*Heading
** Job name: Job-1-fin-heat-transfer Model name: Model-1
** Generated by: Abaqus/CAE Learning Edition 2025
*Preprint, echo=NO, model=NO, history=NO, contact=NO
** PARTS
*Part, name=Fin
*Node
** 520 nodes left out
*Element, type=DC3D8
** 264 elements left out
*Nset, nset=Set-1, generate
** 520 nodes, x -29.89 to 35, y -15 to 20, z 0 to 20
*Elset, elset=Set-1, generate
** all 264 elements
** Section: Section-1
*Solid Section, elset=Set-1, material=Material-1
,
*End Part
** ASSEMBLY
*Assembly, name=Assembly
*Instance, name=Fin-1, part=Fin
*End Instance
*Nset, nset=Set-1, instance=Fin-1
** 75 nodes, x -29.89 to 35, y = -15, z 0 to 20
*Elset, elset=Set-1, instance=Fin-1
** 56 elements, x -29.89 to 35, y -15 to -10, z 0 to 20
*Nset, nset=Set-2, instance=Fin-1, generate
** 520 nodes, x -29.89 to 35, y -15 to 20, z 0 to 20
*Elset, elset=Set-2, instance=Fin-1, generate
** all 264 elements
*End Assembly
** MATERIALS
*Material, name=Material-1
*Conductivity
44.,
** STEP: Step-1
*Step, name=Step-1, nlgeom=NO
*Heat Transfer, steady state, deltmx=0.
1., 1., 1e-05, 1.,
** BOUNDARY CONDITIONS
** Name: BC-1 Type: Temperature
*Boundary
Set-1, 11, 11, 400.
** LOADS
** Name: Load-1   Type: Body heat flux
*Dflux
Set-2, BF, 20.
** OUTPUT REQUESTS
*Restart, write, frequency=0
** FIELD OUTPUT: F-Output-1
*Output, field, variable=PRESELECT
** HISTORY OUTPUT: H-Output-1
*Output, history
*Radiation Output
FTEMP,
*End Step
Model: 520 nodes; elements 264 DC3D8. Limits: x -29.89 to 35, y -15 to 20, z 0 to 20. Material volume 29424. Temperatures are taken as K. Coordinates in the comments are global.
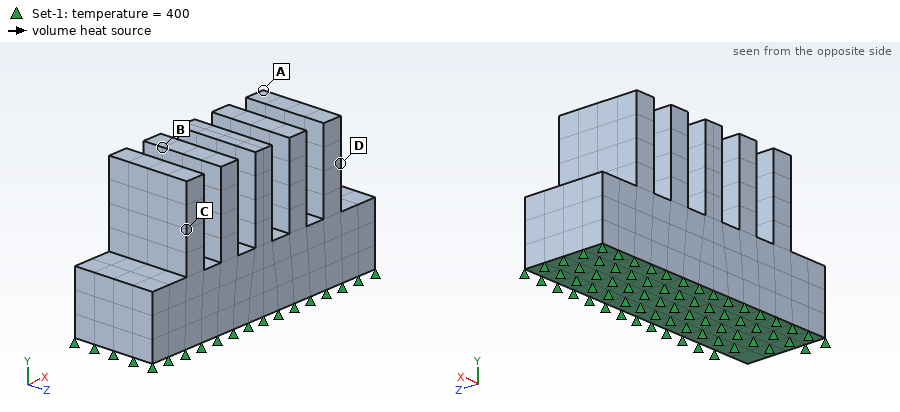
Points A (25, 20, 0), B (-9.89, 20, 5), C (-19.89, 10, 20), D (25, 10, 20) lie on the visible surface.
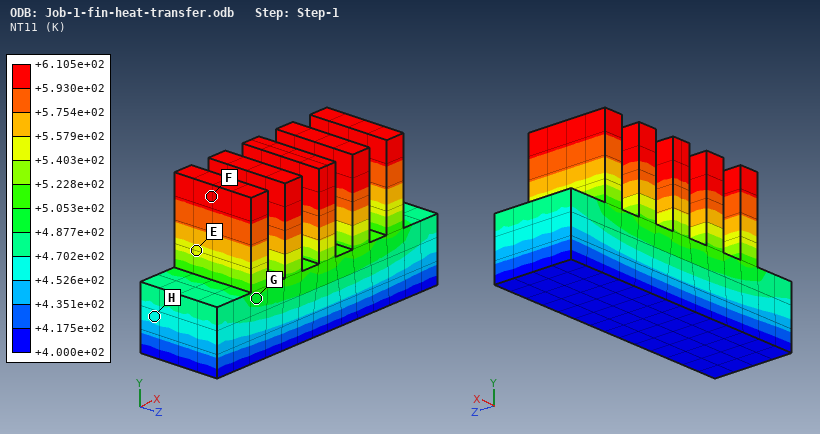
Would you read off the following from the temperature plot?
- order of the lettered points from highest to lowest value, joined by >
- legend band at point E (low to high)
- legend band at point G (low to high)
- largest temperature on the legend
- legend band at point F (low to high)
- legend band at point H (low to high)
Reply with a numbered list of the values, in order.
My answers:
1. F > E > G > H
2. +5.403e+02 to +5.579e+02 K
3. +4.877e+02 to +5.053e+02 K
4. +6.105e+02 K
5. +5.930e+02 to +6.105e+02 K
6. +4.526e+02 to +4.702e+02 K
